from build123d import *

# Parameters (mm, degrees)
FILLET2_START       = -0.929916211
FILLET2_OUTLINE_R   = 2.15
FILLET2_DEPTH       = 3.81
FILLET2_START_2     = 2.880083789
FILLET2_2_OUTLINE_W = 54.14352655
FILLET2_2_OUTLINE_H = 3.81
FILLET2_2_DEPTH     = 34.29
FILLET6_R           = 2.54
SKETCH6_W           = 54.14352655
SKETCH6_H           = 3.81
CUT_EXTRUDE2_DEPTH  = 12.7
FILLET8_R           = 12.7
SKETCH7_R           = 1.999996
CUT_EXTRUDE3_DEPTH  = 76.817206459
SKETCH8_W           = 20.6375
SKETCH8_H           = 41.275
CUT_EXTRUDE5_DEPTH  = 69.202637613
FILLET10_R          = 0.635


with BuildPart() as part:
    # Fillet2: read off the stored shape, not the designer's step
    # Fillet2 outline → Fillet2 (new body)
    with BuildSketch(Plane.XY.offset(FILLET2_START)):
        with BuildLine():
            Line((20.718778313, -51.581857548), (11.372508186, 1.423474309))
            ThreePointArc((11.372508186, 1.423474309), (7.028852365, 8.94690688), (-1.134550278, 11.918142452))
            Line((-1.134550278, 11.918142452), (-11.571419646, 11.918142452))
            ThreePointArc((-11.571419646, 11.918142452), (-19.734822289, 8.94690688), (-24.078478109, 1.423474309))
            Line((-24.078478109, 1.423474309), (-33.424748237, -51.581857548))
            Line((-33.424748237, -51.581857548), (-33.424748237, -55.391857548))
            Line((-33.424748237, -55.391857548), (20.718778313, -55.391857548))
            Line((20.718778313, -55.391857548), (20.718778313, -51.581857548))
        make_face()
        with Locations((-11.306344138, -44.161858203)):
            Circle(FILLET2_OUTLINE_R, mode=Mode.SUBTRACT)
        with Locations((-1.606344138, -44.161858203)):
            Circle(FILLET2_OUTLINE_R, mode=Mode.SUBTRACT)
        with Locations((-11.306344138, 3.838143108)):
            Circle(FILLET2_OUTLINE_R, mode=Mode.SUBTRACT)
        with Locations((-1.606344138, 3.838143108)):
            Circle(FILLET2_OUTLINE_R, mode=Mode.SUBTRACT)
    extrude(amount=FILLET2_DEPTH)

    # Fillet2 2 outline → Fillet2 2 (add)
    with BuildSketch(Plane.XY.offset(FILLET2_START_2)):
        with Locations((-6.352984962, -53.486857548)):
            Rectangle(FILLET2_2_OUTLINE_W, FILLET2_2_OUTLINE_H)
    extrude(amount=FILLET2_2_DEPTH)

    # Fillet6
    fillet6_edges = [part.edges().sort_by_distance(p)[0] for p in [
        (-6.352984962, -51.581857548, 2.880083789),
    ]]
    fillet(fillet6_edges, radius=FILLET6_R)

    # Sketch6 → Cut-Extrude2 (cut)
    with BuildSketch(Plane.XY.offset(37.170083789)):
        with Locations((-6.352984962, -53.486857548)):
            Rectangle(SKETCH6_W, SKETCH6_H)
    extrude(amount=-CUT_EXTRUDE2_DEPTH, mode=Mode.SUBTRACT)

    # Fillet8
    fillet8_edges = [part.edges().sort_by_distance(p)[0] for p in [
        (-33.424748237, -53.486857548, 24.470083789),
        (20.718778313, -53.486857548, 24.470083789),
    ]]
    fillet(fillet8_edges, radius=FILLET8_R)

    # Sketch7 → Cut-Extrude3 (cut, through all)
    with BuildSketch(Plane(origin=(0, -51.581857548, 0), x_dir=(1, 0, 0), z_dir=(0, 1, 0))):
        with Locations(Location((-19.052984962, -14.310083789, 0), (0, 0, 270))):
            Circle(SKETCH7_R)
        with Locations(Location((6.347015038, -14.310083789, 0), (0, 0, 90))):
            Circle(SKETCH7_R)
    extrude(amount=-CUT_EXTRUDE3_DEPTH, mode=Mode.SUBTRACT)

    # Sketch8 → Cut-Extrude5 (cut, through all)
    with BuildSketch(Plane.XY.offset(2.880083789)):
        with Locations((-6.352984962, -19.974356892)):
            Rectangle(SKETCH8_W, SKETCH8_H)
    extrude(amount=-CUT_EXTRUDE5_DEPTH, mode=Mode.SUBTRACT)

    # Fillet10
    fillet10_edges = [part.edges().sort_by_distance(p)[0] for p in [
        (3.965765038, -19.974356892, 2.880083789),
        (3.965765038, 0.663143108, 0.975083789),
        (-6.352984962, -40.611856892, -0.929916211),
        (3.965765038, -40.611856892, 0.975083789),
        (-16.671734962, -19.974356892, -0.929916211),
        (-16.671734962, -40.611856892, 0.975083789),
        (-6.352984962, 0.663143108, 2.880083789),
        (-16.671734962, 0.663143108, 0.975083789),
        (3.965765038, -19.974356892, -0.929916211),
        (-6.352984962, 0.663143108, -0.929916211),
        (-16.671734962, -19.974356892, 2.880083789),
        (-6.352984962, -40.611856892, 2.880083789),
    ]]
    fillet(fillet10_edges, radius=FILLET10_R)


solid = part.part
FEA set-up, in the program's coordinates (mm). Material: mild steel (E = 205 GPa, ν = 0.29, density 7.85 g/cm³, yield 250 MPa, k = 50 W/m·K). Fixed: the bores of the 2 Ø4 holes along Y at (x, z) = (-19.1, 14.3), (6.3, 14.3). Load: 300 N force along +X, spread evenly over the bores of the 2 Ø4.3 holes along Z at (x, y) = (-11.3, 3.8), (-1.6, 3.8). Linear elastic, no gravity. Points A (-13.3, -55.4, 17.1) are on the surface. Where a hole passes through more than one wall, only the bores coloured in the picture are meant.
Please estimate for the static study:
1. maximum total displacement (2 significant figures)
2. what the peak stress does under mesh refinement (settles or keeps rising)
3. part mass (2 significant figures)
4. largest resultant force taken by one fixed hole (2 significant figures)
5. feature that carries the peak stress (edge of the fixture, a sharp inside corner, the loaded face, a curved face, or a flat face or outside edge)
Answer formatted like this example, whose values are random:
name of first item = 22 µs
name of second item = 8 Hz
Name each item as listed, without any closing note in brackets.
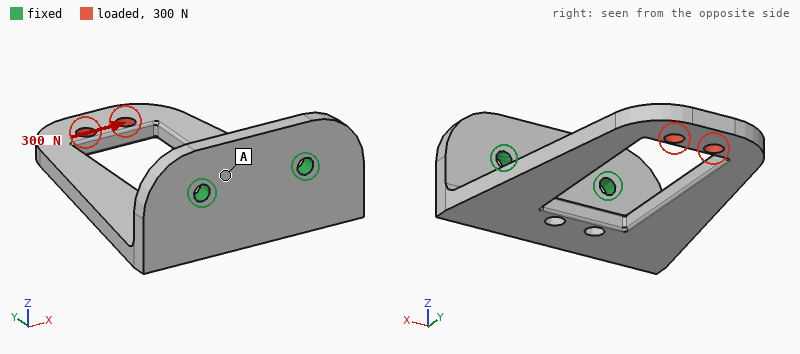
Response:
maximum total displacement = 80 µm
what the peak stress does under mesh refinement = keeps rising
part mass = 92 g
largest resultant force taken by one fixed hole = 580 N
feature that carries the peak stress = edge of the fixture
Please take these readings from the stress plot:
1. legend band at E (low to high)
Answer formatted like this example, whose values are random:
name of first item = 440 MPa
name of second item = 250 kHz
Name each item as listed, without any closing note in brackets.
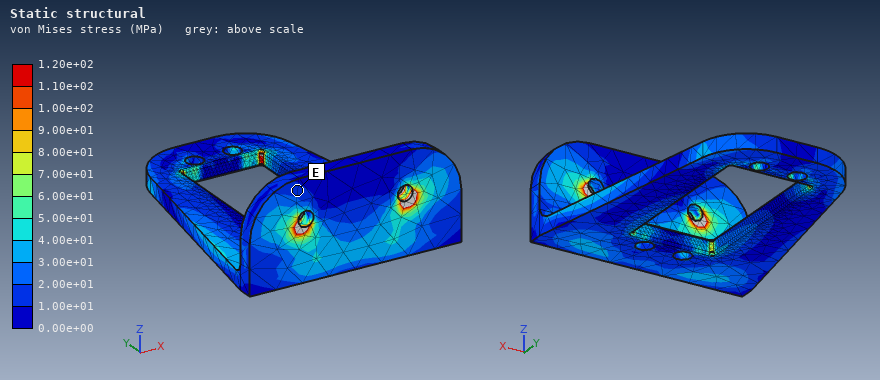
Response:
legend band at E = 1.00e+01 to 2.00e+01 MPa
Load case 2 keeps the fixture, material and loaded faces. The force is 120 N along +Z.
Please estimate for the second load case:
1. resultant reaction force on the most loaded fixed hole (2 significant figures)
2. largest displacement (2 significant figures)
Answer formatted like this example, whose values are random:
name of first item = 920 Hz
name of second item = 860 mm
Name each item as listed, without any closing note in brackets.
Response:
resultant reaction force on the most loaded fixed hole = 63 N
largest displacement = 0.41 mm
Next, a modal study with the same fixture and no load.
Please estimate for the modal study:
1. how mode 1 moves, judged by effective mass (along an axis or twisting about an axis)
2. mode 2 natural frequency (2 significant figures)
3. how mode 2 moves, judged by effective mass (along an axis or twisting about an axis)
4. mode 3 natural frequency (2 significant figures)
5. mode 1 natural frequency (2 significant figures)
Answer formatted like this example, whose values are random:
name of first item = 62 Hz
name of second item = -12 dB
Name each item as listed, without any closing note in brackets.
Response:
how mode 1 moves, judged by effective mass = along Z
mode 2 natural frequency = 2000 Hz
how mode 2 moves, judged by effective mass = along X
mode 3 natural frequency = 2700 Hz
mode 1 natural frequency = 750 Hz
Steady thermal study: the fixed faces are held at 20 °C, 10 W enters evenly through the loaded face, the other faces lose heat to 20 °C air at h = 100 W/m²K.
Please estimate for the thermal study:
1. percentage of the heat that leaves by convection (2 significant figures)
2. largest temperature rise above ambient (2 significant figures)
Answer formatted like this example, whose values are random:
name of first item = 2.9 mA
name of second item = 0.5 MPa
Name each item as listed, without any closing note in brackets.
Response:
percentage of the heat that leaves by convection = 88 %
largest temperature rise above ambient = 67 K
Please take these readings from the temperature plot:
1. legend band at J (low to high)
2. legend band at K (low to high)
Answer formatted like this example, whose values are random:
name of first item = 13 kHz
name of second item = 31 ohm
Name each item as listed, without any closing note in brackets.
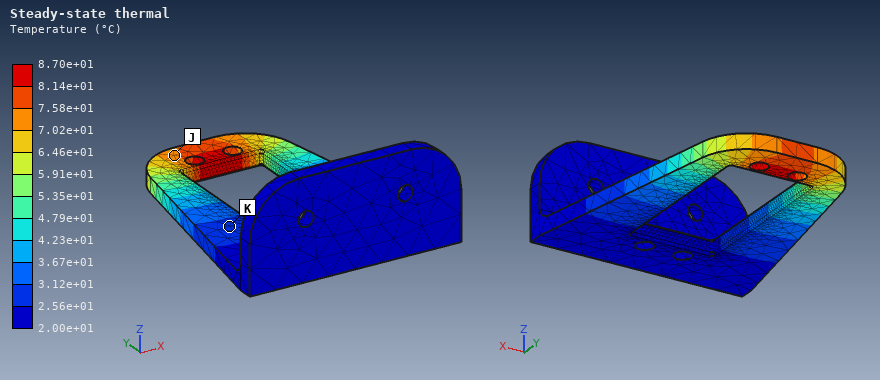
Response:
legend band at J = 7.02e+01 to 7.58e+01 °C
legend band at K = 2.56e+01 to 3.12e+01 °C
